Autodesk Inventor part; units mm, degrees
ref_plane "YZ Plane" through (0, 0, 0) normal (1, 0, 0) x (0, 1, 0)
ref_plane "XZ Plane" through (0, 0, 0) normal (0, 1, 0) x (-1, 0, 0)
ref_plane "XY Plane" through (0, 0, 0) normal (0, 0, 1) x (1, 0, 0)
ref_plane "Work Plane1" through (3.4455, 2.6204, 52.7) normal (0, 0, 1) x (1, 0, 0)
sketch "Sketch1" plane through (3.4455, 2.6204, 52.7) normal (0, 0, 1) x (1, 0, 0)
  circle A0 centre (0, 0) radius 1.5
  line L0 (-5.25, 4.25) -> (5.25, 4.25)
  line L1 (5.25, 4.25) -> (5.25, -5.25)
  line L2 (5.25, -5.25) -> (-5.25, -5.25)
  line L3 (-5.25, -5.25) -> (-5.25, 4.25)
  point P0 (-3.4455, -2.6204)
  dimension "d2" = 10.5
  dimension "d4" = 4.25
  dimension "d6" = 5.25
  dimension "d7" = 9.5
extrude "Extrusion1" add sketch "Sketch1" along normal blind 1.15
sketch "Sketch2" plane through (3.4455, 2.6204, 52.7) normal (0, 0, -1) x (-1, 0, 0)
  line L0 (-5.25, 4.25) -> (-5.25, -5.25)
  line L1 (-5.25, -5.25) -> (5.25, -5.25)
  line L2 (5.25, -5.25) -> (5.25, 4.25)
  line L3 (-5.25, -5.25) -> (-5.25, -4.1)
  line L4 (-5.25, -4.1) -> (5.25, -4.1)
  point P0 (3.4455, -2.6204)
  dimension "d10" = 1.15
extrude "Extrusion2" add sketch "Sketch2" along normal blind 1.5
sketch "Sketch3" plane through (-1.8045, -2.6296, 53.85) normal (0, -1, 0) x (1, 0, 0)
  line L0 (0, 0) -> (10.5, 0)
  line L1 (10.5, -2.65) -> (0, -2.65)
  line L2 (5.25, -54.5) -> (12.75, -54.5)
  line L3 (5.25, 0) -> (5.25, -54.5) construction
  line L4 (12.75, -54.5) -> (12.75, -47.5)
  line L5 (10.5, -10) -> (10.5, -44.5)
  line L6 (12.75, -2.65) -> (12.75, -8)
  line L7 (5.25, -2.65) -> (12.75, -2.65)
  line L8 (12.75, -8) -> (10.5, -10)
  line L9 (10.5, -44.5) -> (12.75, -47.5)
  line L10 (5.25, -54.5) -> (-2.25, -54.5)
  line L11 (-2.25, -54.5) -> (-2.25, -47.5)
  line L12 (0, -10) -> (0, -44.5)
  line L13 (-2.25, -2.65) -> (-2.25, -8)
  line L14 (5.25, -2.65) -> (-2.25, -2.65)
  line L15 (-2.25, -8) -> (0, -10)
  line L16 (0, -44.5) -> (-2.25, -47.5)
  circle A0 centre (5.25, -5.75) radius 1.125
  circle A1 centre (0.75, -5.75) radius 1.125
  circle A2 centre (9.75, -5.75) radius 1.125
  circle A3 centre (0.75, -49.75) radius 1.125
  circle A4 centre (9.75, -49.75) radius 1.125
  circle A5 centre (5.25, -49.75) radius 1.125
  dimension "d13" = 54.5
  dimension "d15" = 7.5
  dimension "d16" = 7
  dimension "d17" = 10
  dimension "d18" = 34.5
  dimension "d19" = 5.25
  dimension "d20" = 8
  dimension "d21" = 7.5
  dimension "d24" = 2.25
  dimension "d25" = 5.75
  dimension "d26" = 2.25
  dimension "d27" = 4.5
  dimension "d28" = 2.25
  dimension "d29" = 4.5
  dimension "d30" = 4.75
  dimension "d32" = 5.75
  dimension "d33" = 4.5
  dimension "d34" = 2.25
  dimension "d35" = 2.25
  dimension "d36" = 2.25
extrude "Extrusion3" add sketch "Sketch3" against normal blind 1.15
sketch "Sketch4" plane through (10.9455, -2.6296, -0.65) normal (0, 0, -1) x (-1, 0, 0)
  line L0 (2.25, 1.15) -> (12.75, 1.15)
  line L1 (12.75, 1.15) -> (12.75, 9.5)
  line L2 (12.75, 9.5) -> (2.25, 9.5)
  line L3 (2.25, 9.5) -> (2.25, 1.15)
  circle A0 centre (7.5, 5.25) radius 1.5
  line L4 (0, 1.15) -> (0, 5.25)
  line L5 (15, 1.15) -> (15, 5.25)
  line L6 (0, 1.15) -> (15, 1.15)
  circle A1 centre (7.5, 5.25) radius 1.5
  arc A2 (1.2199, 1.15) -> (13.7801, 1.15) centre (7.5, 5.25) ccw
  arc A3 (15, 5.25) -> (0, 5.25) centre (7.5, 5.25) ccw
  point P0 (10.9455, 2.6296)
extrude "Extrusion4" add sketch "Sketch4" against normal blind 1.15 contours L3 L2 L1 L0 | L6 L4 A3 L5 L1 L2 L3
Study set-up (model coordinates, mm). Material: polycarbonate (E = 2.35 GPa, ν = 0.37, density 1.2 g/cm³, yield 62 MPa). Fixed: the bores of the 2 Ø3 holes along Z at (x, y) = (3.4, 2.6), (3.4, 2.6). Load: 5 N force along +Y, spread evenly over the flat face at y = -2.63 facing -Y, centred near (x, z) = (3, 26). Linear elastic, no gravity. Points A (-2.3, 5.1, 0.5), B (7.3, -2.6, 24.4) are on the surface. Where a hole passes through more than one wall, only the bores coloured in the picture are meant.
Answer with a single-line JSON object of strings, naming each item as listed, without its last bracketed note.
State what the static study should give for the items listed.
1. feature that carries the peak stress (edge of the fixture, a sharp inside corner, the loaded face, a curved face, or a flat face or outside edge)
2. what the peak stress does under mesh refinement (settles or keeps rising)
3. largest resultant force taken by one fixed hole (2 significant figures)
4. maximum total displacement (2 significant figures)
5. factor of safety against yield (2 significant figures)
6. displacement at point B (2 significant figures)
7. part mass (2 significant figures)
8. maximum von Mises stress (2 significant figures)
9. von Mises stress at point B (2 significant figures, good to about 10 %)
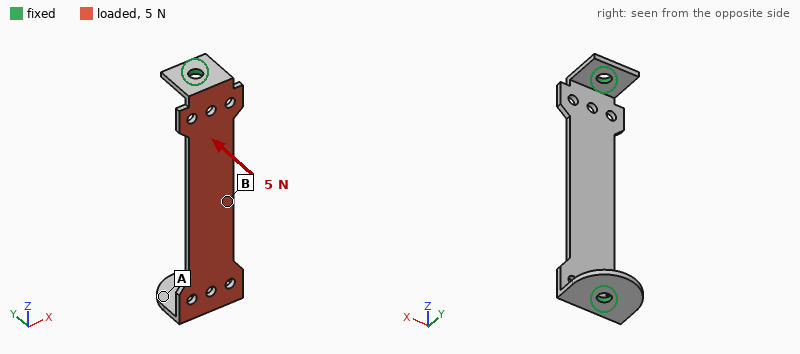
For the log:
{"feature that carries the peak stress": "a curved face", "what the peak stress does under mesh refinement": "settles", "largest resultant force taken by one fixed hole": "6.3 N", "maximum total displacement": "0.65 mm", "factor of safety against yield": "5.4", "displacement at point B": "0.63 mm", "part mass": "1.2 g", "maximum von Mises stress": "12 MPa", "von Mises stress at point B": "5.0 MPa"}
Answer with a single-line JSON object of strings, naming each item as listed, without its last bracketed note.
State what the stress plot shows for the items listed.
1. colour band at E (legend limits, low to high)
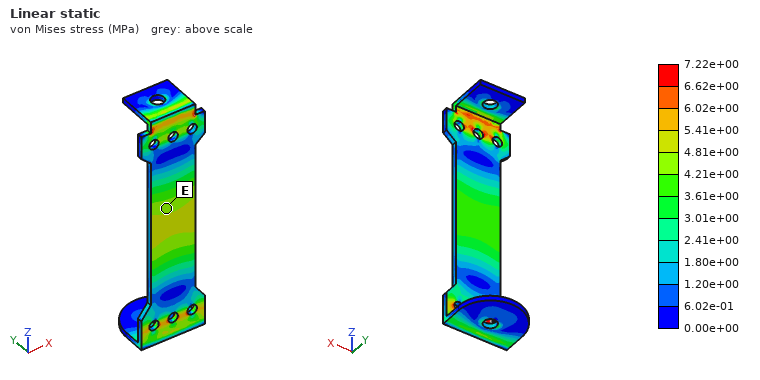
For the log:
{"colour band at E": "4.21e+00 to 4.81e+00 MPa"}
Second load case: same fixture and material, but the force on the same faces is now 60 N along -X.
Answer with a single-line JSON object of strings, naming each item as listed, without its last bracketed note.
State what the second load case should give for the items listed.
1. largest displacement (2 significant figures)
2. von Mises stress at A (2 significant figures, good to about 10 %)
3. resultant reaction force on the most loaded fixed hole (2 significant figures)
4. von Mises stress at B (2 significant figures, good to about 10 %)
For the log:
{"largest displacement": "0.49 mm", "von Mises stress at A": "3.2 MPa", "resultant reaction force on the most loaded fixed hole": "31 N", "von Mises stress at B": "10 MPa"}
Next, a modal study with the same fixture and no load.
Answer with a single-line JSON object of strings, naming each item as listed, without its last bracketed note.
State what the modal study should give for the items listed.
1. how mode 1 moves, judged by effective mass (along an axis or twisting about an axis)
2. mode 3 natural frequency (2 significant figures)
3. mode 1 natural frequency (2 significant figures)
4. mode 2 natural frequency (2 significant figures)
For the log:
{"how mode 1 moves, judged by effective mass": "along Y", "mode 3 natural frequency": "1800 Hz", "mode 1 natural frequency": "560 Hz", "mode 2 natural frequency": "1400 Hz"}
